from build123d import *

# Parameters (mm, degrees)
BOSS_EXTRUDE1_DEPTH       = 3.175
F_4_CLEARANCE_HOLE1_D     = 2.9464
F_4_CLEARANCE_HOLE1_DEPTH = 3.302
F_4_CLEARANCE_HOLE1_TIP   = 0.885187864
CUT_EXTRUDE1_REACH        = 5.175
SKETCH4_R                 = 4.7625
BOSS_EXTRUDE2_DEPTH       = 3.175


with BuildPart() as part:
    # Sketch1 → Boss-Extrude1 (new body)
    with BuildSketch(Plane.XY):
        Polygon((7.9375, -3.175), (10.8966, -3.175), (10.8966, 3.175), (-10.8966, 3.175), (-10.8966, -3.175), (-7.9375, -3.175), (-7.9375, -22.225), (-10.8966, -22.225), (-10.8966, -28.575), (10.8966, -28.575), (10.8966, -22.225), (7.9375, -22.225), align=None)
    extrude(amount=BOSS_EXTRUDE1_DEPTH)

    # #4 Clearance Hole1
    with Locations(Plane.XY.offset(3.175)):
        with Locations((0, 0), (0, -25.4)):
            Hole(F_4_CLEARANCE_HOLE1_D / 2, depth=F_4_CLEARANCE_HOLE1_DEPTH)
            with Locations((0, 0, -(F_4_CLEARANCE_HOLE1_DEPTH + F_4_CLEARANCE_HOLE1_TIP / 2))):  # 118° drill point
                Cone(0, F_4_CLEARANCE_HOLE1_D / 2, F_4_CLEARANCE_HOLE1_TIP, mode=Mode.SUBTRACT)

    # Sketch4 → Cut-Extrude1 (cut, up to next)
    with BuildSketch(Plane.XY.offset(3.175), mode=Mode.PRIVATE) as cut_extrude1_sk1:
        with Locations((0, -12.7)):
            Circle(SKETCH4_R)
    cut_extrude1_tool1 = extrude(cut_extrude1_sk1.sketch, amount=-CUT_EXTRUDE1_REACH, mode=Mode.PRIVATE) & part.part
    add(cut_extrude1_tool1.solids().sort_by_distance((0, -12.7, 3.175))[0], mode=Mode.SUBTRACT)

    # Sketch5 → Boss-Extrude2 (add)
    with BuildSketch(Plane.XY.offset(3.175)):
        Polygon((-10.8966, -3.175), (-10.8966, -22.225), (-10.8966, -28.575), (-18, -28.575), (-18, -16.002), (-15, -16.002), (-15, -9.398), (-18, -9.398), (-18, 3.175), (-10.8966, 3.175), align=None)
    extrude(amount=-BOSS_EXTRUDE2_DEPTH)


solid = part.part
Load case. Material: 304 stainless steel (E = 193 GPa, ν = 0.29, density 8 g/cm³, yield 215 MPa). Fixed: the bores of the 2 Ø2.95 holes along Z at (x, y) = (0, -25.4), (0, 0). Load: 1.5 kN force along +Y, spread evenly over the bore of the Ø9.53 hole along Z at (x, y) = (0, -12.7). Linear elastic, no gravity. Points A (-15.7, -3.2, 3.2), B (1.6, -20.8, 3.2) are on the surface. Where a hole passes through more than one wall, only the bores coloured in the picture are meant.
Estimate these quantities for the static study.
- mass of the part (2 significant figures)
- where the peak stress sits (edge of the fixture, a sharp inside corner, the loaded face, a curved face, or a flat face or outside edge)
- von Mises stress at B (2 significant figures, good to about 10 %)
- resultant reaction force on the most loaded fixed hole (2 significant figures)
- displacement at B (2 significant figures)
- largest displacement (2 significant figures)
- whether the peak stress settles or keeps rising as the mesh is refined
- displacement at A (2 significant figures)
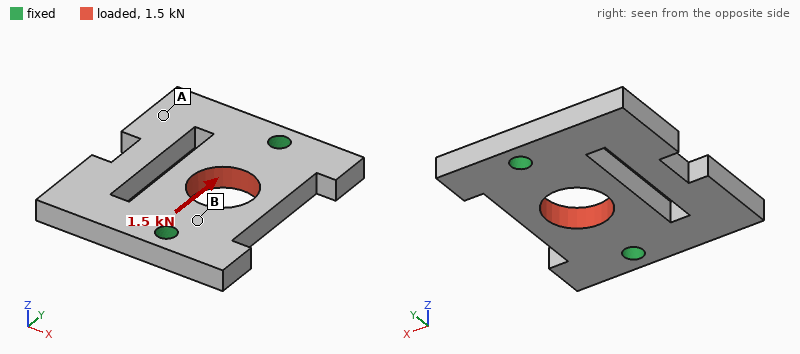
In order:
18 g
edge of the fixture
27 MPa
750 N
0.62 µm
1.6 µm
keeps rising
1.2 µm
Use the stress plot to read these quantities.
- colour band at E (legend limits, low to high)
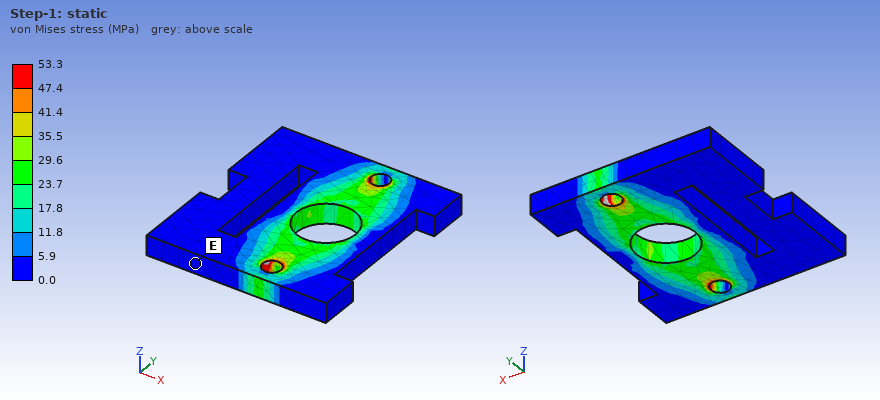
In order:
0.0 to 5.9 MPa
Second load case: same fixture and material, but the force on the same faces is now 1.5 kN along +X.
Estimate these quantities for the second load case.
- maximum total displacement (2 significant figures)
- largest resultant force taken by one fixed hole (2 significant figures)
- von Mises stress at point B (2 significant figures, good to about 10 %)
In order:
4.2 µm
750 N
34 MPa
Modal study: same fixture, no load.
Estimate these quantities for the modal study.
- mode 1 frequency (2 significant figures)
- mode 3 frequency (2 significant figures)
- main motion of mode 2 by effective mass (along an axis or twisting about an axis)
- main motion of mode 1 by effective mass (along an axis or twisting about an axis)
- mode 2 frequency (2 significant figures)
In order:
6300 Hz
19 kHz
twisting about X
along Z
11 kHz
